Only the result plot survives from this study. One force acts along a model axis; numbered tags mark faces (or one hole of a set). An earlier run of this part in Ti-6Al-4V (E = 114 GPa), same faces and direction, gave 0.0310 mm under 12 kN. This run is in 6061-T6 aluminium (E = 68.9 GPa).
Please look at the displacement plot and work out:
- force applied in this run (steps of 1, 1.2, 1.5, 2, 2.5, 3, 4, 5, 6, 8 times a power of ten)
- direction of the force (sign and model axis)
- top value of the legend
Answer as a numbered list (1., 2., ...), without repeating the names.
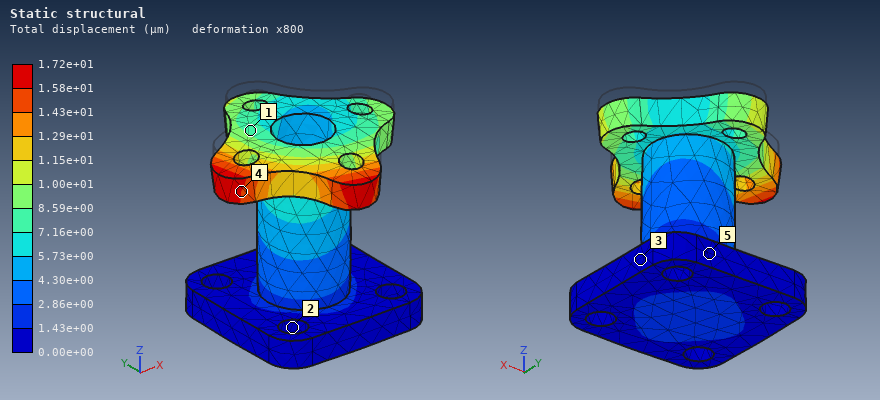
1. 4 kN
2. -Z
3. 1.72e+01 µm
